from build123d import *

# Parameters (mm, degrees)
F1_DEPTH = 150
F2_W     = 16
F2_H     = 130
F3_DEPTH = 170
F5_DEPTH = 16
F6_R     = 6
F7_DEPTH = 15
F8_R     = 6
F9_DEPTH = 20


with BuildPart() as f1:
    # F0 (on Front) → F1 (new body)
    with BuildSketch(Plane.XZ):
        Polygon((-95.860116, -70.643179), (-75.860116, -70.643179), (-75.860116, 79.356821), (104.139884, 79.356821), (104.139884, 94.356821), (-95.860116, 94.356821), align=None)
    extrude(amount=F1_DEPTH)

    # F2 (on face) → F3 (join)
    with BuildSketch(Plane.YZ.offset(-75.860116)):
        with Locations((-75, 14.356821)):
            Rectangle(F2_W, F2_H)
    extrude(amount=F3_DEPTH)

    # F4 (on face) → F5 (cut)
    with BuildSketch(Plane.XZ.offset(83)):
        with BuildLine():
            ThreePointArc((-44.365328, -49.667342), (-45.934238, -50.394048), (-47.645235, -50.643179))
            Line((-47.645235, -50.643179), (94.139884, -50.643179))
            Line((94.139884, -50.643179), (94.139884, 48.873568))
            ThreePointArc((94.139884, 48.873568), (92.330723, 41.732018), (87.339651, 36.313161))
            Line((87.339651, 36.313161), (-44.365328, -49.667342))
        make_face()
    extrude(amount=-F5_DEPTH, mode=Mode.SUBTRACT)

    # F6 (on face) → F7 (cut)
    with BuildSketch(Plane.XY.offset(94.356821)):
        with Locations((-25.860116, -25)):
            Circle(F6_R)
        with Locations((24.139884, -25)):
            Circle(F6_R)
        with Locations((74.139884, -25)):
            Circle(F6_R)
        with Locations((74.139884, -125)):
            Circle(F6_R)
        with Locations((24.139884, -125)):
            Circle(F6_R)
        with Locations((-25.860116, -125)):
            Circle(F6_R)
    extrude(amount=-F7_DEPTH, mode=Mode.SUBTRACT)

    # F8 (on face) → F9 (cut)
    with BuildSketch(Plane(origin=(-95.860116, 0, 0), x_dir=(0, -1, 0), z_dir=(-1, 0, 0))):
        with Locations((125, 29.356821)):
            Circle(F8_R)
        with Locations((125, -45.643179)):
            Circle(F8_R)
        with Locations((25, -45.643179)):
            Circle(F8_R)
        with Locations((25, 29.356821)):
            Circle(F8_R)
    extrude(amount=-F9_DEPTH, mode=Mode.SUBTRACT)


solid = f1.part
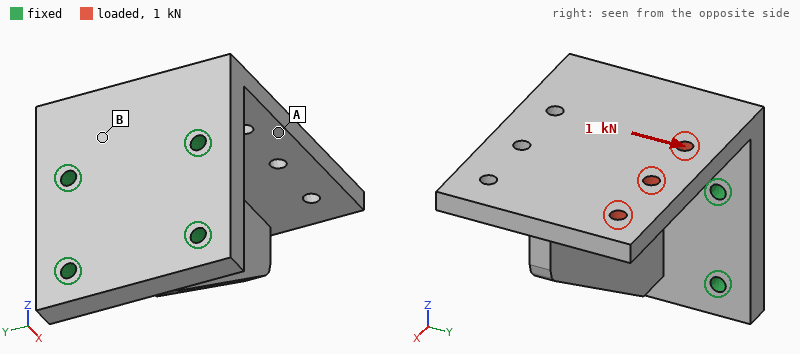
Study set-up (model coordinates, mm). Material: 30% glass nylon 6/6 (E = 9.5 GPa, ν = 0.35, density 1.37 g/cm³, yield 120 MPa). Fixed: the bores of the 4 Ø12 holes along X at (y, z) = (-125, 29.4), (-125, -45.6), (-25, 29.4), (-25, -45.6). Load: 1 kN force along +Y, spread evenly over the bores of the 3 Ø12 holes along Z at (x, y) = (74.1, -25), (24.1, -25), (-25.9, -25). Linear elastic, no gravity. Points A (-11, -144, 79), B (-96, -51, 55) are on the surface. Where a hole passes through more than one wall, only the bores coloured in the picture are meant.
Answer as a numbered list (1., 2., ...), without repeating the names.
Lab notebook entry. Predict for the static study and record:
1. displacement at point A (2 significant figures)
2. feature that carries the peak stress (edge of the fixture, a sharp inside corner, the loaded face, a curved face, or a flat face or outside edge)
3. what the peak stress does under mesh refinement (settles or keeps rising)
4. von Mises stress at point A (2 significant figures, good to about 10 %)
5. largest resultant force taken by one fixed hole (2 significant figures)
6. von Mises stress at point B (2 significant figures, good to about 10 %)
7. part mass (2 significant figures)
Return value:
1. 0.16 mm
2. edge of the fixture
3. keeps rising
4. 0.94 MPa
5. 1.3 kN
6. 2.5 MPa
7. 1.6 kg
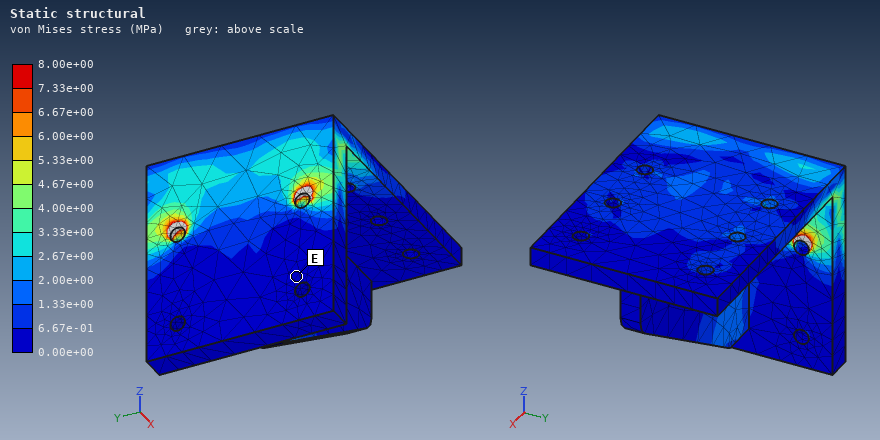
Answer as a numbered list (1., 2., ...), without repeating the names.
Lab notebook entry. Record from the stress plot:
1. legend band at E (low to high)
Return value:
1. 0.00e+00 to 6.67e-01 MPa
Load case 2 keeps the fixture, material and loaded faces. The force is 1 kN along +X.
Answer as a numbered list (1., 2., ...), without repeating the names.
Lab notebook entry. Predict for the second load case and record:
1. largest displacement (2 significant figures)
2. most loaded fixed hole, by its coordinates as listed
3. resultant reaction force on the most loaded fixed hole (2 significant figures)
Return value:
1. 0.19 mm
2. (-25, 29.4)
3. 1.2 kN
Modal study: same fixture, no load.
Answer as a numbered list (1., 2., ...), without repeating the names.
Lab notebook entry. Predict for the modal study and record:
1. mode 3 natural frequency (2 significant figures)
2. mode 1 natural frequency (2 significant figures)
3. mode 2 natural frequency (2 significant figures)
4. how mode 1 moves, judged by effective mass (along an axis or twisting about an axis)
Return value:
1. 620 Hz
2. 410 Hz
3. 520 Hz
4. along Y
